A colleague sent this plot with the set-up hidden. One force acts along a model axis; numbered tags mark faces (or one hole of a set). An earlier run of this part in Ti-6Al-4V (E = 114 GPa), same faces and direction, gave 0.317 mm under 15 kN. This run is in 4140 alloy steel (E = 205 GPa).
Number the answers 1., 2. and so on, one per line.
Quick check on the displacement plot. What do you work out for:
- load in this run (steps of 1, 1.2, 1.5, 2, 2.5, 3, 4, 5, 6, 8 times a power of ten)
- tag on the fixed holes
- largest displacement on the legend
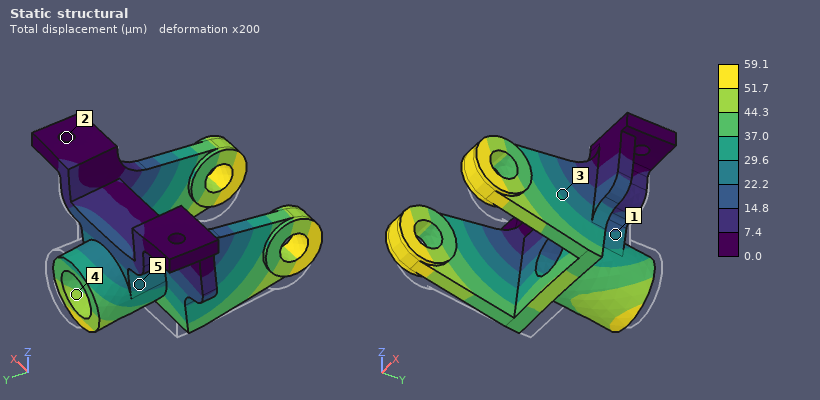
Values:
1. 5 kN
2. 2
3. 59.1 µm
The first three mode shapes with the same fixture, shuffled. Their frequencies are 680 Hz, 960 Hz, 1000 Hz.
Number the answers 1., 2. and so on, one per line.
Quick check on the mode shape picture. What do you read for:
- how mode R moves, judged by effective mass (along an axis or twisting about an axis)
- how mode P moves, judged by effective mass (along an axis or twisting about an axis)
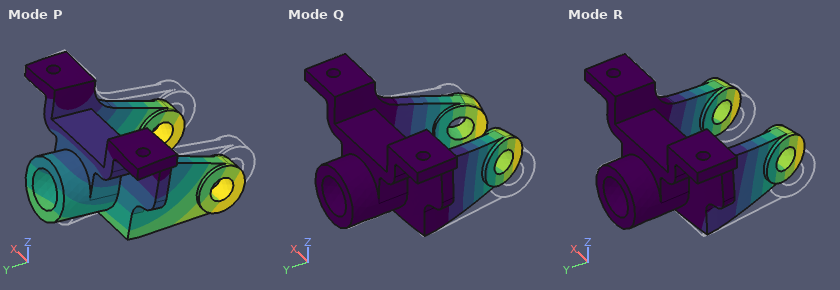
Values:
1. along X
2. along Y
